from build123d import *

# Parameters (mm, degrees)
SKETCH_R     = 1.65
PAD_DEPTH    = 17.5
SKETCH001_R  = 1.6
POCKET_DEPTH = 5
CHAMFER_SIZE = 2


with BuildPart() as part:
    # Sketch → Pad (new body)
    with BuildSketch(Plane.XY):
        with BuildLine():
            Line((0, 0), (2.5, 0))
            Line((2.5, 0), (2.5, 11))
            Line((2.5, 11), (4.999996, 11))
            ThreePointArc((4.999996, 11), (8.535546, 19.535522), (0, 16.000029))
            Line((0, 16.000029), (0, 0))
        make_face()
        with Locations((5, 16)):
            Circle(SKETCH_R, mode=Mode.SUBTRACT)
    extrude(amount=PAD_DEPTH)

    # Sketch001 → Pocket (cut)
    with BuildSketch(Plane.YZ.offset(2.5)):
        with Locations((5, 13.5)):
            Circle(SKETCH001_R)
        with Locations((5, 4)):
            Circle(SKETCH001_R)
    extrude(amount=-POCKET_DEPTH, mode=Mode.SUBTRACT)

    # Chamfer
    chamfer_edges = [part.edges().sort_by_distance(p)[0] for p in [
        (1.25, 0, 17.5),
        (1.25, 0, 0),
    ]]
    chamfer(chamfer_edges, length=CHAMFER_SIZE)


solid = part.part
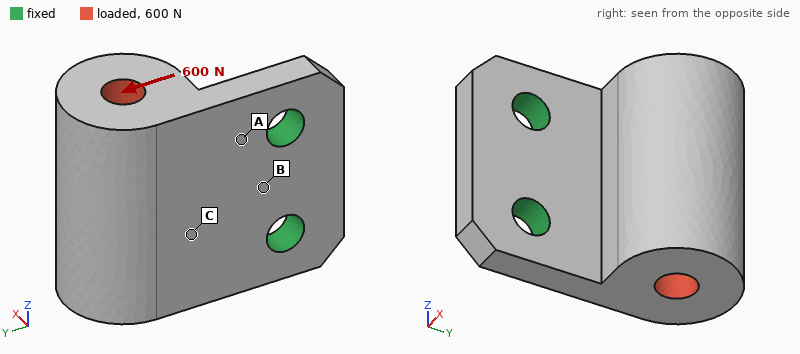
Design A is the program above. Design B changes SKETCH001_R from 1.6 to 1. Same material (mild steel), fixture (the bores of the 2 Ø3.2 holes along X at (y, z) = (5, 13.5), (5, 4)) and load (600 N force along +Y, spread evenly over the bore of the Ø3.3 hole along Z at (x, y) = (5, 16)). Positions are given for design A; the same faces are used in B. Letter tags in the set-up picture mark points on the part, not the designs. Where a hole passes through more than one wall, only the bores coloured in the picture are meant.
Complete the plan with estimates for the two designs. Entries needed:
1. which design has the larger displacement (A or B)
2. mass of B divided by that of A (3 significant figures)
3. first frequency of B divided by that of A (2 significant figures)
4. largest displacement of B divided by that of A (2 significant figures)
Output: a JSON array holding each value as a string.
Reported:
["B", "1.01", "0.90", "1.2"]
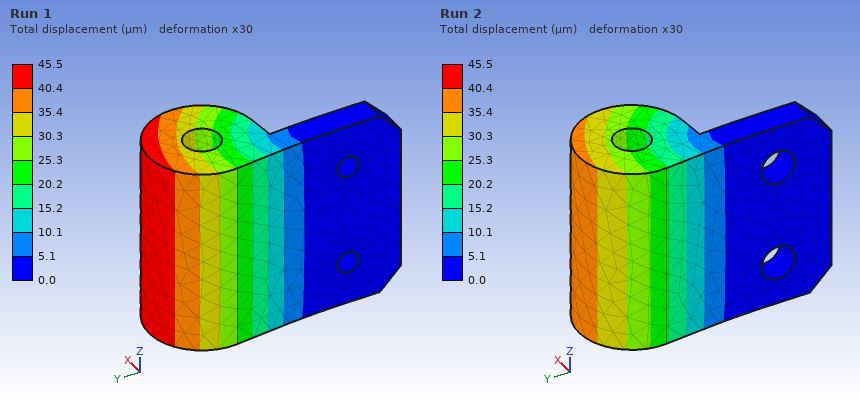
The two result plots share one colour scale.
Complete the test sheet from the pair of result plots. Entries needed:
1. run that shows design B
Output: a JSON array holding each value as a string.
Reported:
["Run 1"]
